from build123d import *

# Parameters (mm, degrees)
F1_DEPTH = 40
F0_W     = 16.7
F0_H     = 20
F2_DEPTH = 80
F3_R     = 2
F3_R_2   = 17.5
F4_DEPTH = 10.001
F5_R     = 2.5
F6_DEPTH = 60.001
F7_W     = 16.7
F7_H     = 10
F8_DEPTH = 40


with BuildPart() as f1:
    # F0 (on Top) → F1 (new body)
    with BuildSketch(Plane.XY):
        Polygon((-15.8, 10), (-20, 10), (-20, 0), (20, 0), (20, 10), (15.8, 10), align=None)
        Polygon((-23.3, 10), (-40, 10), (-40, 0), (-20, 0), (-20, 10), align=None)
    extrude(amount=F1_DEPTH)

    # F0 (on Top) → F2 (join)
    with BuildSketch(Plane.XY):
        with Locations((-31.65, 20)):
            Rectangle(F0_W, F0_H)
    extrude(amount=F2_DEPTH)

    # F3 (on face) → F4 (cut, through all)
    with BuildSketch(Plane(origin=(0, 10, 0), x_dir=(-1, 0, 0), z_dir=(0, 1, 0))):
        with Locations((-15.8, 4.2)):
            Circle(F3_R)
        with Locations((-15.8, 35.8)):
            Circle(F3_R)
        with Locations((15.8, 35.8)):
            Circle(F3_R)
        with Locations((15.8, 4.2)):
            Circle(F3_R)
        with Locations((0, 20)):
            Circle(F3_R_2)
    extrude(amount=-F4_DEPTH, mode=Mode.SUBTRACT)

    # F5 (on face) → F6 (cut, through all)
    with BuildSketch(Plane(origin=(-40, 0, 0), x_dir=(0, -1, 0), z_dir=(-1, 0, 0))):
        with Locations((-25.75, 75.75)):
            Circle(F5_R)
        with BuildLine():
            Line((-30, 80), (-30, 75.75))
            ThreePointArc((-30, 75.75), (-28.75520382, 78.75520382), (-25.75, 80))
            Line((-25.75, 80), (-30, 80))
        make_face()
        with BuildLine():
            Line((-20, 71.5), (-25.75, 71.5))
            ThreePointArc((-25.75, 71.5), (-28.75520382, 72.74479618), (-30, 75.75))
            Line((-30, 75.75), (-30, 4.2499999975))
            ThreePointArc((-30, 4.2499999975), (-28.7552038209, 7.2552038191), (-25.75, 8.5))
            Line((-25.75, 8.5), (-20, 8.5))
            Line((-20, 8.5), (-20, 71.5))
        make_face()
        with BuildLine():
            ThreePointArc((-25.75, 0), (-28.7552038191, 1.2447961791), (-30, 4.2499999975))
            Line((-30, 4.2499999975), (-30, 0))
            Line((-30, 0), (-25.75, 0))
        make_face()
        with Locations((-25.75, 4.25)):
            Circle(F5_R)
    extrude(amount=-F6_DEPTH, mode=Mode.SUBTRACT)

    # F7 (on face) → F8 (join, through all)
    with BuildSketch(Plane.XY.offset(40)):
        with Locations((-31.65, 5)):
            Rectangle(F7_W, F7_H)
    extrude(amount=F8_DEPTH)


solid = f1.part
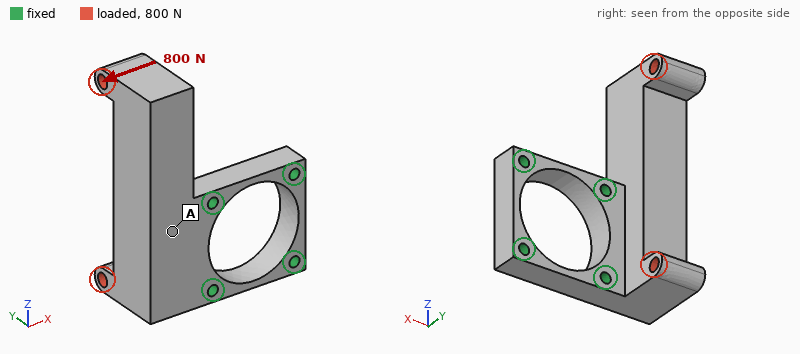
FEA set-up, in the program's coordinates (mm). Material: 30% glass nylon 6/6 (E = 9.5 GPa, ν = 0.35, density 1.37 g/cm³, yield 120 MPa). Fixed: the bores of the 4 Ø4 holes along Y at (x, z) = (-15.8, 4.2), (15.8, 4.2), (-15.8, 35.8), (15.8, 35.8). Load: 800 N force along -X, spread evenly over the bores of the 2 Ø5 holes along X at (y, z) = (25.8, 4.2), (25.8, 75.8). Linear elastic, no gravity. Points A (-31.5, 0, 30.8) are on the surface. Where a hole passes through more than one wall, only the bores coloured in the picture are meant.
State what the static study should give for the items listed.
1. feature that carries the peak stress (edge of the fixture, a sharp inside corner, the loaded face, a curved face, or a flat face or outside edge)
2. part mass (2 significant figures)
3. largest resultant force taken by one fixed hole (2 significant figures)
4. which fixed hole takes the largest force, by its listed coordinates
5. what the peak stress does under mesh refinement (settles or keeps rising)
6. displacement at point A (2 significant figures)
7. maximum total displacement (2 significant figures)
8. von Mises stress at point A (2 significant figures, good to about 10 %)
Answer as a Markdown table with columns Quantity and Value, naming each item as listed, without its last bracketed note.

| Quantity | Value |
|---|---|
| feature that carries the peak stress | edge of the fixture |
| part mass | 49 g |
| largest resultant force taken by one fixed hole | 920 N |
| which fixed hole takes the largest force, by its listed coordinates | (-15.8, 35.8) |
| what the peak stress does under mesh refinement | keeps rising |
| displacement at point A | 0.11 mm |
| maximum total displacement | 0.61 mm |
| von Mises stress at point A | 11 MPa |
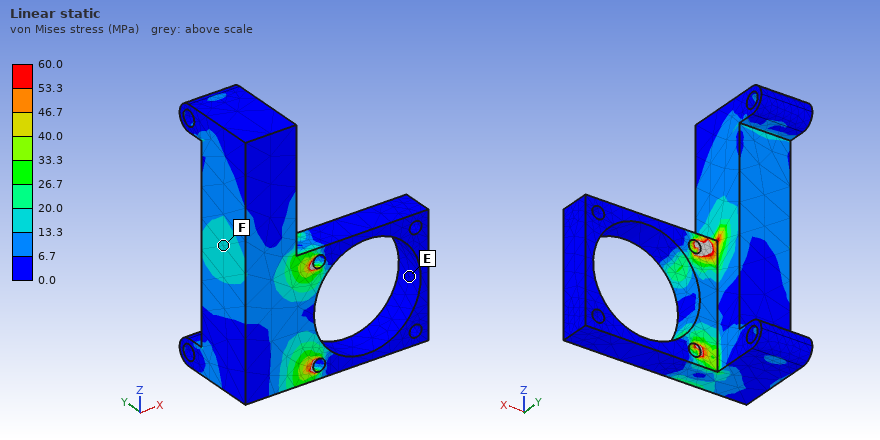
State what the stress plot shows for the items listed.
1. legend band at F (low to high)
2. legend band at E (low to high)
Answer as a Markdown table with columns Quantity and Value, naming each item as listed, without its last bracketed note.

| Quantity | Value |
|---|---|
| legend band at F | 13.3 to 20.0 MPa |
| legend band at E | 0.0 to 6.7 MPa |
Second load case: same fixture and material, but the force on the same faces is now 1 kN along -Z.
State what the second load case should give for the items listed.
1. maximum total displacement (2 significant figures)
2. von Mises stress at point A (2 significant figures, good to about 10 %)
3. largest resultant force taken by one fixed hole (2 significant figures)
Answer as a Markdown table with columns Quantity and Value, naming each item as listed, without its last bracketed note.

| Quantity | Value |
|---|---|
| maximum total displacement | 0.30 mm |
| von Mises stress at point A | 5.2 MPa |
| largest resultant force taken by one fixed hole | 910 N |
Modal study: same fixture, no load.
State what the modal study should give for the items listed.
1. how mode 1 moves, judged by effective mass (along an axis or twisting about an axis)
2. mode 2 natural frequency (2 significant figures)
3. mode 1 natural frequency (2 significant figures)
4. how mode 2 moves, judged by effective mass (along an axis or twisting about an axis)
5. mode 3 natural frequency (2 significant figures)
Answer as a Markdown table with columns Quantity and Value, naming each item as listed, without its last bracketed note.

| Quantity | Value |
|---|---|
| how mode 1 moves, judged by effective mass | along Y |
| mode 2 natural frequency | 2300 Hz |
| mode 1 natural frequency | 1600 Hz |
| how mode 2 moves, judged by effective mass | along X |
| mode 3 natural frequency | 2900 Hz |
